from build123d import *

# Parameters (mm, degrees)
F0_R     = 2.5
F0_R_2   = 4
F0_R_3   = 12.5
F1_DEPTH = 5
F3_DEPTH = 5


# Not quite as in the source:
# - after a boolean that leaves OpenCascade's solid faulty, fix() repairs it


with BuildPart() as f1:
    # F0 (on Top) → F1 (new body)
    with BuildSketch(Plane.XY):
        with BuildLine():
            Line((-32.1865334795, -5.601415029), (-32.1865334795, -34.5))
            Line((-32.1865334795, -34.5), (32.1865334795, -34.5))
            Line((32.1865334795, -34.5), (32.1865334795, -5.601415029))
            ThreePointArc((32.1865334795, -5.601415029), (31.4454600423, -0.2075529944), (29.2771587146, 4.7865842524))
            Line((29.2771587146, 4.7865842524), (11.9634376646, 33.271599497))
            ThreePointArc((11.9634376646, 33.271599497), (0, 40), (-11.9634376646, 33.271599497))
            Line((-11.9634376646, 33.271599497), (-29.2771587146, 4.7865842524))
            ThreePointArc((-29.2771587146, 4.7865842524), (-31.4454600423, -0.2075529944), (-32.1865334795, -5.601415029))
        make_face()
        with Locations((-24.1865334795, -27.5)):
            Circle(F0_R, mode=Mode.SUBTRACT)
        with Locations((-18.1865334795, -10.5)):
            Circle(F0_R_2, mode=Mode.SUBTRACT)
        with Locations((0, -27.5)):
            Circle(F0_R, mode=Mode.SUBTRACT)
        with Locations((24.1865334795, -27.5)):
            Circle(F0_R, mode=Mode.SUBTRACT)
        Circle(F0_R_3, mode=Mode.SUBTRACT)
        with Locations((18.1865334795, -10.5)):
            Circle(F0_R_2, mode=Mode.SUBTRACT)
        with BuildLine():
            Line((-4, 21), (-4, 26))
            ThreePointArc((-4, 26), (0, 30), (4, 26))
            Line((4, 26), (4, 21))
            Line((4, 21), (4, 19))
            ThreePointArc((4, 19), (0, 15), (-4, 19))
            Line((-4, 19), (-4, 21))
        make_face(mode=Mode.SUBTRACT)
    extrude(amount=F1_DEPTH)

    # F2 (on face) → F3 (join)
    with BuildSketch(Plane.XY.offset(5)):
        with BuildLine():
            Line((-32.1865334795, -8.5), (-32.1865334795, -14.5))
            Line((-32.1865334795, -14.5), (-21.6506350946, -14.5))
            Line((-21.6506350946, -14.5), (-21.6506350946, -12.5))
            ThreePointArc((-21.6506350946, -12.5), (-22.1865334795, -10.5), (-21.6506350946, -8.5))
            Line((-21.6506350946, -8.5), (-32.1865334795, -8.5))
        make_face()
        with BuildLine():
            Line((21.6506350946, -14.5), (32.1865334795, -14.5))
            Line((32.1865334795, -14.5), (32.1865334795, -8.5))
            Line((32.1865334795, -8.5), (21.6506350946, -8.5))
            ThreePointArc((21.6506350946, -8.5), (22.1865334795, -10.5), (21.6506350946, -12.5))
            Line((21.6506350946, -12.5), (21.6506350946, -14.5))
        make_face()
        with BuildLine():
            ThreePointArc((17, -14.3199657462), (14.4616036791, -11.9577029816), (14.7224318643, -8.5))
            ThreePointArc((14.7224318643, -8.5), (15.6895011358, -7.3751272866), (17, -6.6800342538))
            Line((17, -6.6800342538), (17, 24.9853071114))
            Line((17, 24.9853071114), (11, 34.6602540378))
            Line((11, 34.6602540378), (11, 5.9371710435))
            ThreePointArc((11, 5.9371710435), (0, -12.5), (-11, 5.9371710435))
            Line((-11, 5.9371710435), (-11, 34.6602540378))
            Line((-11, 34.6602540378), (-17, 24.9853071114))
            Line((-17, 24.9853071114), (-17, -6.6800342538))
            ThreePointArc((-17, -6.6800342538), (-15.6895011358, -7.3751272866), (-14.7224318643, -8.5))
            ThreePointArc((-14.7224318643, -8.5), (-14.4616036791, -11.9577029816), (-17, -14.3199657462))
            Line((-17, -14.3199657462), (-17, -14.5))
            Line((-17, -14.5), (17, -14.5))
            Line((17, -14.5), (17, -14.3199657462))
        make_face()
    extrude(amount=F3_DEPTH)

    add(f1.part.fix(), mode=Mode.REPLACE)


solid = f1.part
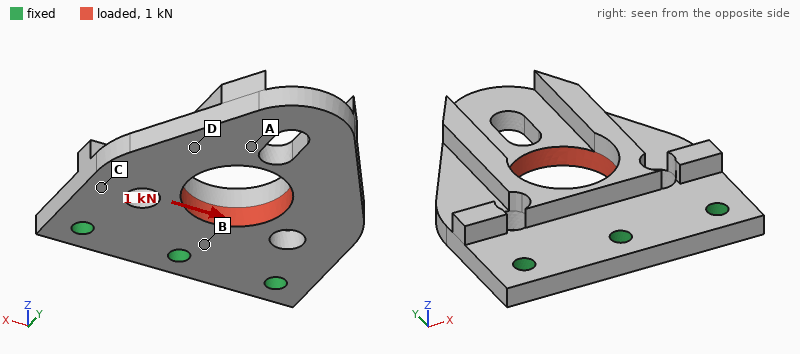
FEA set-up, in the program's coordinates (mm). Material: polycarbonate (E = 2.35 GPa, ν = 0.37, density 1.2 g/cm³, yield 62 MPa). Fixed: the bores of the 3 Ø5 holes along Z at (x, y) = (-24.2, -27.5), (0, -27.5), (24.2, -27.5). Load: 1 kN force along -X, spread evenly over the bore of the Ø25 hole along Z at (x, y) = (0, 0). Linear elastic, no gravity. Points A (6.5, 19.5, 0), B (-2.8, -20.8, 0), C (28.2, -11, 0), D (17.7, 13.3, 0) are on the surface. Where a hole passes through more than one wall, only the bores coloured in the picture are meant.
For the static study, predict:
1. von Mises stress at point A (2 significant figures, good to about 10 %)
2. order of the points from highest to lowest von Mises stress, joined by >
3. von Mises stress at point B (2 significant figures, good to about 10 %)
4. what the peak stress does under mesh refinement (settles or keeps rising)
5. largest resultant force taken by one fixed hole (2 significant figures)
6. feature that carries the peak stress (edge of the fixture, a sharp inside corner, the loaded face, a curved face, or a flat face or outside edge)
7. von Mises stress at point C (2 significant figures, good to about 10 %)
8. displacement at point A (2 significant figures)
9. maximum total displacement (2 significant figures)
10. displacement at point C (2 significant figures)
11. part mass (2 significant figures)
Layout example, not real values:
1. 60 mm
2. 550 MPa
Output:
1. 4.3 MPa
2. B > C > A > D
3. 10 MPa
4. keeps rising
5. 570 N
6. edge of the fixture
7. 7.8 MPa
8. 0.37 mm
9. 0.40 mm
10. 0.14 mm
11. 22 g
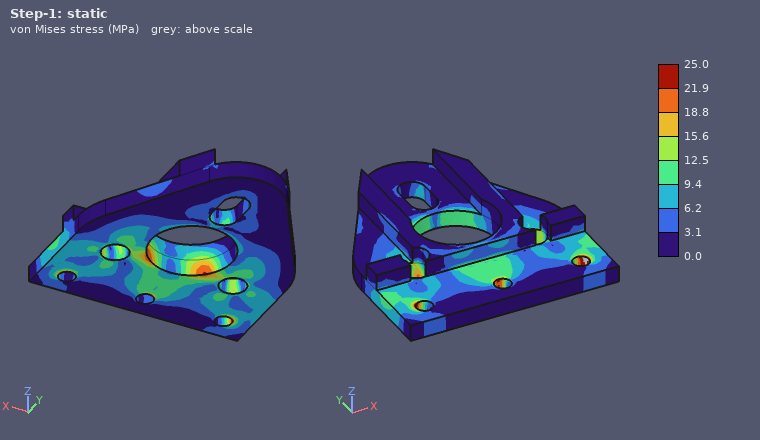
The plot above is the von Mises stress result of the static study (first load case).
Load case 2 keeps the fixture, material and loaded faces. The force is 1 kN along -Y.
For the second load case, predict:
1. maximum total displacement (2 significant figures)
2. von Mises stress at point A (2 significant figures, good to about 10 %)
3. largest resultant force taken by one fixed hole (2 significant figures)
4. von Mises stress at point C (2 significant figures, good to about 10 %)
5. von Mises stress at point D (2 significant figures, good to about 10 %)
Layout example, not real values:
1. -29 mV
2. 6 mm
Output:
1. 0.32 mm
2. 2.8 MPa
3. 350 N
4. 4.3 MPa
5. 2.9 MPa
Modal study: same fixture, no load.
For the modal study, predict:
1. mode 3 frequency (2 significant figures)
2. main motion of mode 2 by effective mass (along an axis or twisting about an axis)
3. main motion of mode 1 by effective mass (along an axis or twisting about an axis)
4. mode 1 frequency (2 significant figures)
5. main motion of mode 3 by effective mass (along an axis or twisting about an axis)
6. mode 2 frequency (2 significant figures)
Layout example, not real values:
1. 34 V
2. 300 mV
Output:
1. 2000 Hz
2. twisting about Y
3. along Z
4. 360 Hz
5. along X
6. 1000 Hz
